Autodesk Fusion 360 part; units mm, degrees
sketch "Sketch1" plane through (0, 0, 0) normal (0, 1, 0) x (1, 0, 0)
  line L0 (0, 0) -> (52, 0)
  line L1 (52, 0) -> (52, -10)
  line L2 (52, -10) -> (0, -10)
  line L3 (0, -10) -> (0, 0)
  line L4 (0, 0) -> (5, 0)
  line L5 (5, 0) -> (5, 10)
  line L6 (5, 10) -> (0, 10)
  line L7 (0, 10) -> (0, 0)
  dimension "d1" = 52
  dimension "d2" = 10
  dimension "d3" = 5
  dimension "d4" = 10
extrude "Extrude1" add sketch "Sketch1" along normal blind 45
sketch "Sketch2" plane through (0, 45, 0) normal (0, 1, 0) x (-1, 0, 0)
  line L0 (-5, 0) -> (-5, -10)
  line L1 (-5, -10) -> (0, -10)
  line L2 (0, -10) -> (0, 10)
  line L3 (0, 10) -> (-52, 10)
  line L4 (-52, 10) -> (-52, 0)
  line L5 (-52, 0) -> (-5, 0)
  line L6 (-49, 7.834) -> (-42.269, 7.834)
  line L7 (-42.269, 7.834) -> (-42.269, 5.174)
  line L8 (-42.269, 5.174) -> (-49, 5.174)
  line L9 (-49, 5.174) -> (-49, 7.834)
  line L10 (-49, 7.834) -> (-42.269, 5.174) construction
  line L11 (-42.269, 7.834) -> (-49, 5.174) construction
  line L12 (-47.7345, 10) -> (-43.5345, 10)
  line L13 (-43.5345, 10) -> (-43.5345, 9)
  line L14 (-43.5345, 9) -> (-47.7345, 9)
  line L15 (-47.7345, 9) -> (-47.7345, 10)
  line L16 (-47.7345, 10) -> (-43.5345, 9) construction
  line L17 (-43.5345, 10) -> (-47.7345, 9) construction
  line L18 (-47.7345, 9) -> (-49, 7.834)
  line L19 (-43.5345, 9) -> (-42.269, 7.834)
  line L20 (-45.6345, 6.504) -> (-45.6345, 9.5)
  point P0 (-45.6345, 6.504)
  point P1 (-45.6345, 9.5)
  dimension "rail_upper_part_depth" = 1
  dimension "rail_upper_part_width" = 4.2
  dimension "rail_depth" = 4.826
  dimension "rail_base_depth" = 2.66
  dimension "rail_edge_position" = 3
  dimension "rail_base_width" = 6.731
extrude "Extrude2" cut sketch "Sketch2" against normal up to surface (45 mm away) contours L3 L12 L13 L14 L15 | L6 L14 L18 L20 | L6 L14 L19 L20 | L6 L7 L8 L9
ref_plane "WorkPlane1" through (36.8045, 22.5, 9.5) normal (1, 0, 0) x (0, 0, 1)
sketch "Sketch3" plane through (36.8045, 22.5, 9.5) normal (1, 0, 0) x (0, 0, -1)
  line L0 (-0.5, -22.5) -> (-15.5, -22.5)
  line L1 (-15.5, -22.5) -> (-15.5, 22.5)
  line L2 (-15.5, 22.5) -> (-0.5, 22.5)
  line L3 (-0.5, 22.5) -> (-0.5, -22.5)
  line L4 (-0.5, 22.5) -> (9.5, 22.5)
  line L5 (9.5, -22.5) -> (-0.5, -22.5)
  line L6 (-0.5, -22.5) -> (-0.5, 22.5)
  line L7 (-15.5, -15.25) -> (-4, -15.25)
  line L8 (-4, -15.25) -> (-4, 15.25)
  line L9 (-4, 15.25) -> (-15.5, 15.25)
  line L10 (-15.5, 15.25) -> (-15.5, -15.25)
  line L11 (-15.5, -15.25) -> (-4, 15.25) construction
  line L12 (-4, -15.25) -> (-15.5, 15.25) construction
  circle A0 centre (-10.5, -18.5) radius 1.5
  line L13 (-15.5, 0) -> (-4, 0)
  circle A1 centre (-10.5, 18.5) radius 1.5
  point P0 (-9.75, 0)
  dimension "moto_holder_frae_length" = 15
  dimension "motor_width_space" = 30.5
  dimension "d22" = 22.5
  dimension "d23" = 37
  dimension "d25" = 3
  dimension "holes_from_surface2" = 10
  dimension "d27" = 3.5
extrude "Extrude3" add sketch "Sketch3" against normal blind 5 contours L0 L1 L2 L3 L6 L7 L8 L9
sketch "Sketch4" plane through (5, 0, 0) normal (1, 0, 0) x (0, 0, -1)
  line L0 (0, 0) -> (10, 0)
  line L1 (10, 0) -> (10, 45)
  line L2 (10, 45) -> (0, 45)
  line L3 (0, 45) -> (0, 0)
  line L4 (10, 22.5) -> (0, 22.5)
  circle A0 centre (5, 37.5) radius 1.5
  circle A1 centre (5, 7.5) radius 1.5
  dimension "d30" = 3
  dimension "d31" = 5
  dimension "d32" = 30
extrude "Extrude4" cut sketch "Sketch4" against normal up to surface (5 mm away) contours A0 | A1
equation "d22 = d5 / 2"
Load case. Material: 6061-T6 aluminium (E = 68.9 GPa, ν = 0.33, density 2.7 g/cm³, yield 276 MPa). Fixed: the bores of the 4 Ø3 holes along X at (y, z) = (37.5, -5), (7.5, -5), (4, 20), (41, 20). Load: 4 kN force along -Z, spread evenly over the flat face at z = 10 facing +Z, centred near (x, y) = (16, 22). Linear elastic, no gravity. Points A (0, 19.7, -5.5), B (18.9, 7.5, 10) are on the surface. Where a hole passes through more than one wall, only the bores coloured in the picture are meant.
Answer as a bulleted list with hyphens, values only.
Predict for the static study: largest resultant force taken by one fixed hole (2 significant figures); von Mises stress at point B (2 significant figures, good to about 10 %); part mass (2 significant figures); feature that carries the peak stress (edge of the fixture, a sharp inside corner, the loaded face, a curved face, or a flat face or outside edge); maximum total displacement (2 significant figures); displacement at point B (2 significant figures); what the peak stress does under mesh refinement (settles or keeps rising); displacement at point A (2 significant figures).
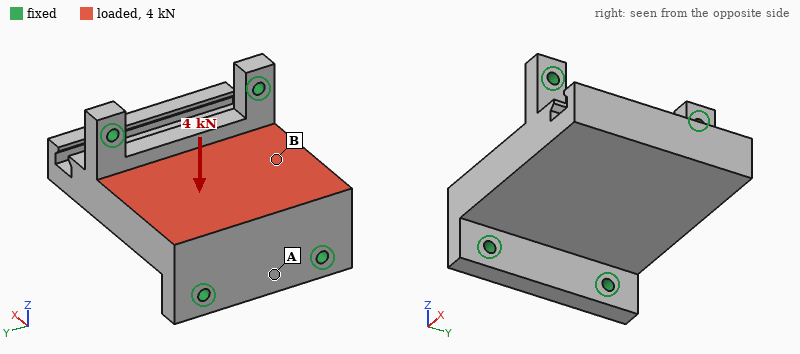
- 1.2 kN
- 16 MPa
- 70 g
- edge of the fixture
- 12 µm
- 11 µm
- keeps rising
- 2.5 µm
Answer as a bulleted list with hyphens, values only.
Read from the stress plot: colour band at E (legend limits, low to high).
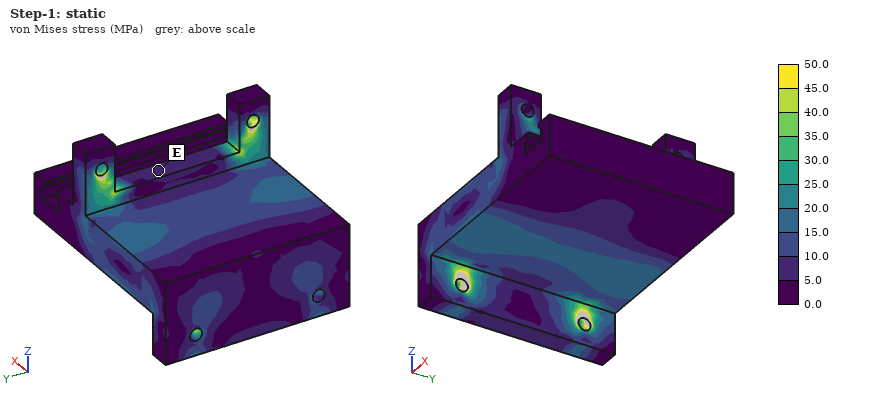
- 5.0 to 10.0 MPa
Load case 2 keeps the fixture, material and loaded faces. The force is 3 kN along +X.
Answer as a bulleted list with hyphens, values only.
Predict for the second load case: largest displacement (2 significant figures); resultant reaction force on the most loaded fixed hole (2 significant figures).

- 18 µm
- 1.2 kN
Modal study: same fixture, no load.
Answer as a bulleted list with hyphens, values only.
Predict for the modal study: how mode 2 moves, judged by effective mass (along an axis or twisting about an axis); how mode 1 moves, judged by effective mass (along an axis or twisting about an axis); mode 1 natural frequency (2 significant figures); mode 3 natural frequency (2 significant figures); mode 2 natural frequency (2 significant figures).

- along X
- along Y
- 8300 Hz
- 11 kHz
- 8800 Hz
